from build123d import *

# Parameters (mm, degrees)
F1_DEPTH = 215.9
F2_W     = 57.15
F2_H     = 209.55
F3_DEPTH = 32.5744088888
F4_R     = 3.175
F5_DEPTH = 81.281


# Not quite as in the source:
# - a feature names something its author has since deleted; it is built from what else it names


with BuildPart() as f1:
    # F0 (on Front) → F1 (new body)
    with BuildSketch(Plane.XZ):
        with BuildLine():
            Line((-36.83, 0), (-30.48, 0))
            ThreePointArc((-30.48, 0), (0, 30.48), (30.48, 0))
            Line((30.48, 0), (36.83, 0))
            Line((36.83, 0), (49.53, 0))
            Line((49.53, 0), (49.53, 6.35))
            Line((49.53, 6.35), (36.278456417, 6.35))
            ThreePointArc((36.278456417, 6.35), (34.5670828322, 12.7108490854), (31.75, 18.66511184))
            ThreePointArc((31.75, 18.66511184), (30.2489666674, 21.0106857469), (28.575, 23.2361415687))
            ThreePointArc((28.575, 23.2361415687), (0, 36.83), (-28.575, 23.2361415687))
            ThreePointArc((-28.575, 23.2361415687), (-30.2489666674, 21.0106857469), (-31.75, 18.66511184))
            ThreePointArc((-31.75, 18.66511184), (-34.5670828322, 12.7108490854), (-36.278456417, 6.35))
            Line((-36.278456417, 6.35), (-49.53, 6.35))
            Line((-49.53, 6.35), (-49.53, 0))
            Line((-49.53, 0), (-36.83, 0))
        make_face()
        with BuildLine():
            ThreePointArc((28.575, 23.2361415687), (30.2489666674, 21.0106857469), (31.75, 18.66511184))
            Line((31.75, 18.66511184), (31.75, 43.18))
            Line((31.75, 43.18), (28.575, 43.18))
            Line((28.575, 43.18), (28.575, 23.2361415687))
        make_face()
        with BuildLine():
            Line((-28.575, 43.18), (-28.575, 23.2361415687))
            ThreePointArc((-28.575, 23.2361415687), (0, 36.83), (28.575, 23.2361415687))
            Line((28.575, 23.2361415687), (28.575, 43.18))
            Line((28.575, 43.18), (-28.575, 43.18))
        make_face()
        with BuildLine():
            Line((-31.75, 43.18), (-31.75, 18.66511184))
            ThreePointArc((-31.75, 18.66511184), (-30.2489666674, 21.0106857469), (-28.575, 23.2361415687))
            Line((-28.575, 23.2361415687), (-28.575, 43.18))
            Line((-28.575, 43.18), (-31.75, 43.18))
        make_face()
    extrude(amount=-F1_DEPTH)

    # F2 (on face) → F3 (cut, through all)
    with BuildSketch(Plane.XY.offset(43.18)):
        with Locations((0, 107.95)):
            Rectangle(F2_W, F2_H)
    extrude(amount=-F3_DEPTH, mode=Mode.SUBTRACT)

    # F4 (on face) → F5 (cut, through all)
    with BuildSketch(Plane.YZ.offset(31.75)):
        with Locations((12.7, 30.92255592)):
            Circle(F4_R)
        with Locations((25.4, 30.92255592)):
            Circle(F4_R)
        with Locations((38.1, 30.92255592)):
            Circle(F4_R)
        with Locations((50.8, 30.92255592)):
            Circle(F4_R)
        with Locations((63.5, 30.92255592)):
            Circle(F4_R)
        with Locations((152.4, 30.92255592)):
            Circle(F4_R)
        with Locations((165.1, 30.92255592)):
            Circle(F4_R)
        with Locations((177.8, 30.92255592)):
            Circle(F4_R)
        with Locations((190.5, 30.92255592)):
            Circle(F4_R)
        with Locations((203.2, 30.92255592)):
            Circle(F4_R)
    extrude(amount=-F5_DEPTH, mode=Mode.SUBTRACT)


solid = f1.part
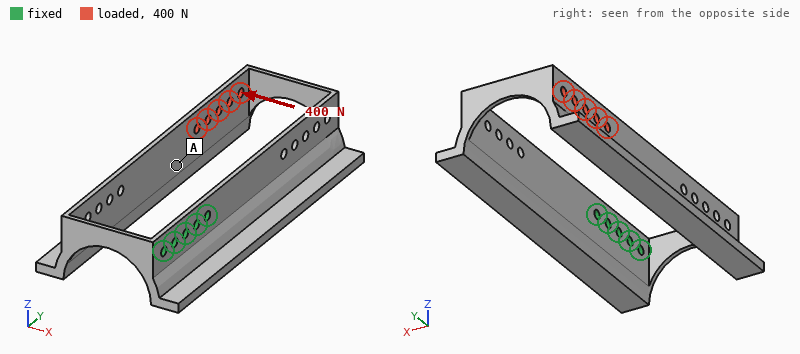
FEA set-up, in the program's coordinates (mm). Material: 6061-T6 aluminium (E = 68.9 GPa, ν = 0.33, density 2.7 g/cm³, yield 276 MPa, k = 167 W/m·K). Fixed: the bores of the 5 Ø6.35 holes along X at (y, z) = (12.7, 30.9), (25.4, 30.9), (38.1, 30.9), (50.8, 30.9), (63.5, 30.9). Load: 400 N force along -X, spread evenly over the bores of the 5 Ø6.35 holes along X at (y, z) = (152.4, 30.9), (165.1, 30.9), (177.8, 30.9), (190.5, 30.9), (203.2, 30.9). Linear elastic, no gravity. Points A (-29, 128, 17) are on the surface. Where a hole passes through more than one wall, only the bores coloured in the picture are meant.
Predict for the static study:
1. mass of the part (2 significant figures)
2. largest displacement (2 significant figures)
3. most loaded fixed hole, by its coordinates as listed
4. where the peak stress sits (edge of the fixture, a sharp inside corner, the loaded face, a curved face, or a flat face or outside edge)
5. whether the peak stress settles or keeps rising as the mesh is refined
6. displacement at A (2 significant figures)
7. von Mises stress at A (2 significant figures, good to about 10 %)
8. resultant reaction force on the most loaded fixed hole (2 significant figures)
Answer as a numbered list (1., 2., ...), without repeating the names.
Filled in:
1. 330 g
2. 2.8 mm
3. (63.5, 30.9)
4. edge of the fixture
5. keeps rising
6. 1.7 mm
7. 13 MPa
8. 1.2 kN
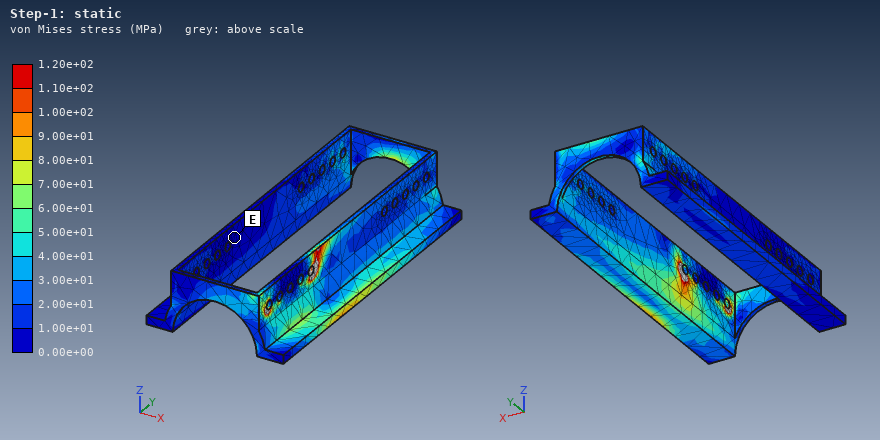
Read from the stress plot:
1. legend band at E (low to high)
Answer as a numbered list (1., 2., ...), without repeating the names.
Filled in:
1. 0.00e+00 to 1.00e+01 MPa
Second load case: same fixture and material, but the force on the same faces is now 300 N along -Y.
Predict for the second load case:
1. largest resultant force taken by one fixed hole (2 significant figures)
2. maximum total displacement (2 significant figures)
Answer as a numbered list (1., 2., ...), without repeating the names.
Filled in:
1. 270 N
2. 1.6 mm
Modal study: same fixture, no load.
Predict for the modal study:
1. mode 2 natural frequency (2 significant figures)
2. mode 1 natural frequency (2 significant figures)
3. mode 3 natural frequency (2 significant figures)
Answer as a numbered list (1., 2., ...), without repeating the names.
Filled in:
1. 180 Hz
2. 150 Hz
3. 240 Hz
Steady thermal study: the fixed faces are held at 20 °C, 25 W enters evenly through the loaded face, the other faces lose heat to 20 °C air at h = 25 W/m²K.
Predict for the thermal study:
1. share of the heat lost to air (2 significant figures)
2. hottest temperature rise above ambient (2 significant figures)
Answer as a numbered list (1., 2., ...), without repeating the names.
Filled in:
1. 88 %
2. 48 K
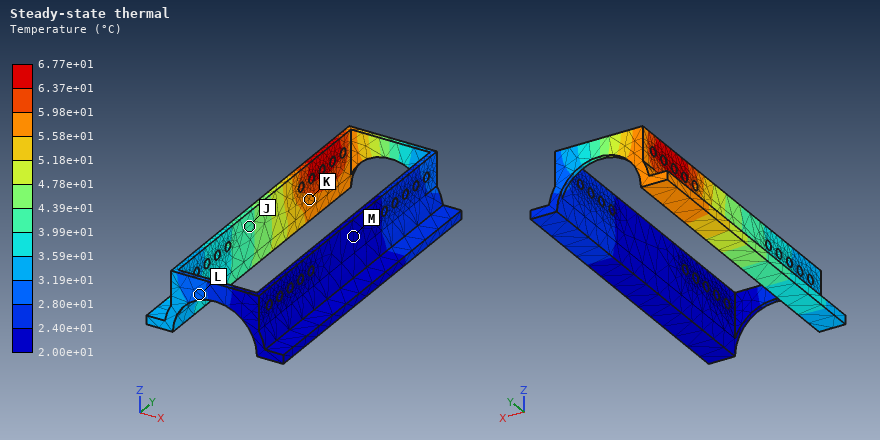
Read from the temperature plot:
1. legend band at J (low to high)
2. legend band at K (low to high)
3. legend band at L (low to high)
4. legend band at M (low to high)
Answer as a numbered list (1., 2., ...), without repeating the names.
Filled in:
1. 3.99e+01 to 4.39e+01 °C
2. 5.58e+01 to 5.98e+01 °C
3. 2.80e+01 to 3.19e+01 °C
4. 2.00e+01 to 2.40e+01 °C
